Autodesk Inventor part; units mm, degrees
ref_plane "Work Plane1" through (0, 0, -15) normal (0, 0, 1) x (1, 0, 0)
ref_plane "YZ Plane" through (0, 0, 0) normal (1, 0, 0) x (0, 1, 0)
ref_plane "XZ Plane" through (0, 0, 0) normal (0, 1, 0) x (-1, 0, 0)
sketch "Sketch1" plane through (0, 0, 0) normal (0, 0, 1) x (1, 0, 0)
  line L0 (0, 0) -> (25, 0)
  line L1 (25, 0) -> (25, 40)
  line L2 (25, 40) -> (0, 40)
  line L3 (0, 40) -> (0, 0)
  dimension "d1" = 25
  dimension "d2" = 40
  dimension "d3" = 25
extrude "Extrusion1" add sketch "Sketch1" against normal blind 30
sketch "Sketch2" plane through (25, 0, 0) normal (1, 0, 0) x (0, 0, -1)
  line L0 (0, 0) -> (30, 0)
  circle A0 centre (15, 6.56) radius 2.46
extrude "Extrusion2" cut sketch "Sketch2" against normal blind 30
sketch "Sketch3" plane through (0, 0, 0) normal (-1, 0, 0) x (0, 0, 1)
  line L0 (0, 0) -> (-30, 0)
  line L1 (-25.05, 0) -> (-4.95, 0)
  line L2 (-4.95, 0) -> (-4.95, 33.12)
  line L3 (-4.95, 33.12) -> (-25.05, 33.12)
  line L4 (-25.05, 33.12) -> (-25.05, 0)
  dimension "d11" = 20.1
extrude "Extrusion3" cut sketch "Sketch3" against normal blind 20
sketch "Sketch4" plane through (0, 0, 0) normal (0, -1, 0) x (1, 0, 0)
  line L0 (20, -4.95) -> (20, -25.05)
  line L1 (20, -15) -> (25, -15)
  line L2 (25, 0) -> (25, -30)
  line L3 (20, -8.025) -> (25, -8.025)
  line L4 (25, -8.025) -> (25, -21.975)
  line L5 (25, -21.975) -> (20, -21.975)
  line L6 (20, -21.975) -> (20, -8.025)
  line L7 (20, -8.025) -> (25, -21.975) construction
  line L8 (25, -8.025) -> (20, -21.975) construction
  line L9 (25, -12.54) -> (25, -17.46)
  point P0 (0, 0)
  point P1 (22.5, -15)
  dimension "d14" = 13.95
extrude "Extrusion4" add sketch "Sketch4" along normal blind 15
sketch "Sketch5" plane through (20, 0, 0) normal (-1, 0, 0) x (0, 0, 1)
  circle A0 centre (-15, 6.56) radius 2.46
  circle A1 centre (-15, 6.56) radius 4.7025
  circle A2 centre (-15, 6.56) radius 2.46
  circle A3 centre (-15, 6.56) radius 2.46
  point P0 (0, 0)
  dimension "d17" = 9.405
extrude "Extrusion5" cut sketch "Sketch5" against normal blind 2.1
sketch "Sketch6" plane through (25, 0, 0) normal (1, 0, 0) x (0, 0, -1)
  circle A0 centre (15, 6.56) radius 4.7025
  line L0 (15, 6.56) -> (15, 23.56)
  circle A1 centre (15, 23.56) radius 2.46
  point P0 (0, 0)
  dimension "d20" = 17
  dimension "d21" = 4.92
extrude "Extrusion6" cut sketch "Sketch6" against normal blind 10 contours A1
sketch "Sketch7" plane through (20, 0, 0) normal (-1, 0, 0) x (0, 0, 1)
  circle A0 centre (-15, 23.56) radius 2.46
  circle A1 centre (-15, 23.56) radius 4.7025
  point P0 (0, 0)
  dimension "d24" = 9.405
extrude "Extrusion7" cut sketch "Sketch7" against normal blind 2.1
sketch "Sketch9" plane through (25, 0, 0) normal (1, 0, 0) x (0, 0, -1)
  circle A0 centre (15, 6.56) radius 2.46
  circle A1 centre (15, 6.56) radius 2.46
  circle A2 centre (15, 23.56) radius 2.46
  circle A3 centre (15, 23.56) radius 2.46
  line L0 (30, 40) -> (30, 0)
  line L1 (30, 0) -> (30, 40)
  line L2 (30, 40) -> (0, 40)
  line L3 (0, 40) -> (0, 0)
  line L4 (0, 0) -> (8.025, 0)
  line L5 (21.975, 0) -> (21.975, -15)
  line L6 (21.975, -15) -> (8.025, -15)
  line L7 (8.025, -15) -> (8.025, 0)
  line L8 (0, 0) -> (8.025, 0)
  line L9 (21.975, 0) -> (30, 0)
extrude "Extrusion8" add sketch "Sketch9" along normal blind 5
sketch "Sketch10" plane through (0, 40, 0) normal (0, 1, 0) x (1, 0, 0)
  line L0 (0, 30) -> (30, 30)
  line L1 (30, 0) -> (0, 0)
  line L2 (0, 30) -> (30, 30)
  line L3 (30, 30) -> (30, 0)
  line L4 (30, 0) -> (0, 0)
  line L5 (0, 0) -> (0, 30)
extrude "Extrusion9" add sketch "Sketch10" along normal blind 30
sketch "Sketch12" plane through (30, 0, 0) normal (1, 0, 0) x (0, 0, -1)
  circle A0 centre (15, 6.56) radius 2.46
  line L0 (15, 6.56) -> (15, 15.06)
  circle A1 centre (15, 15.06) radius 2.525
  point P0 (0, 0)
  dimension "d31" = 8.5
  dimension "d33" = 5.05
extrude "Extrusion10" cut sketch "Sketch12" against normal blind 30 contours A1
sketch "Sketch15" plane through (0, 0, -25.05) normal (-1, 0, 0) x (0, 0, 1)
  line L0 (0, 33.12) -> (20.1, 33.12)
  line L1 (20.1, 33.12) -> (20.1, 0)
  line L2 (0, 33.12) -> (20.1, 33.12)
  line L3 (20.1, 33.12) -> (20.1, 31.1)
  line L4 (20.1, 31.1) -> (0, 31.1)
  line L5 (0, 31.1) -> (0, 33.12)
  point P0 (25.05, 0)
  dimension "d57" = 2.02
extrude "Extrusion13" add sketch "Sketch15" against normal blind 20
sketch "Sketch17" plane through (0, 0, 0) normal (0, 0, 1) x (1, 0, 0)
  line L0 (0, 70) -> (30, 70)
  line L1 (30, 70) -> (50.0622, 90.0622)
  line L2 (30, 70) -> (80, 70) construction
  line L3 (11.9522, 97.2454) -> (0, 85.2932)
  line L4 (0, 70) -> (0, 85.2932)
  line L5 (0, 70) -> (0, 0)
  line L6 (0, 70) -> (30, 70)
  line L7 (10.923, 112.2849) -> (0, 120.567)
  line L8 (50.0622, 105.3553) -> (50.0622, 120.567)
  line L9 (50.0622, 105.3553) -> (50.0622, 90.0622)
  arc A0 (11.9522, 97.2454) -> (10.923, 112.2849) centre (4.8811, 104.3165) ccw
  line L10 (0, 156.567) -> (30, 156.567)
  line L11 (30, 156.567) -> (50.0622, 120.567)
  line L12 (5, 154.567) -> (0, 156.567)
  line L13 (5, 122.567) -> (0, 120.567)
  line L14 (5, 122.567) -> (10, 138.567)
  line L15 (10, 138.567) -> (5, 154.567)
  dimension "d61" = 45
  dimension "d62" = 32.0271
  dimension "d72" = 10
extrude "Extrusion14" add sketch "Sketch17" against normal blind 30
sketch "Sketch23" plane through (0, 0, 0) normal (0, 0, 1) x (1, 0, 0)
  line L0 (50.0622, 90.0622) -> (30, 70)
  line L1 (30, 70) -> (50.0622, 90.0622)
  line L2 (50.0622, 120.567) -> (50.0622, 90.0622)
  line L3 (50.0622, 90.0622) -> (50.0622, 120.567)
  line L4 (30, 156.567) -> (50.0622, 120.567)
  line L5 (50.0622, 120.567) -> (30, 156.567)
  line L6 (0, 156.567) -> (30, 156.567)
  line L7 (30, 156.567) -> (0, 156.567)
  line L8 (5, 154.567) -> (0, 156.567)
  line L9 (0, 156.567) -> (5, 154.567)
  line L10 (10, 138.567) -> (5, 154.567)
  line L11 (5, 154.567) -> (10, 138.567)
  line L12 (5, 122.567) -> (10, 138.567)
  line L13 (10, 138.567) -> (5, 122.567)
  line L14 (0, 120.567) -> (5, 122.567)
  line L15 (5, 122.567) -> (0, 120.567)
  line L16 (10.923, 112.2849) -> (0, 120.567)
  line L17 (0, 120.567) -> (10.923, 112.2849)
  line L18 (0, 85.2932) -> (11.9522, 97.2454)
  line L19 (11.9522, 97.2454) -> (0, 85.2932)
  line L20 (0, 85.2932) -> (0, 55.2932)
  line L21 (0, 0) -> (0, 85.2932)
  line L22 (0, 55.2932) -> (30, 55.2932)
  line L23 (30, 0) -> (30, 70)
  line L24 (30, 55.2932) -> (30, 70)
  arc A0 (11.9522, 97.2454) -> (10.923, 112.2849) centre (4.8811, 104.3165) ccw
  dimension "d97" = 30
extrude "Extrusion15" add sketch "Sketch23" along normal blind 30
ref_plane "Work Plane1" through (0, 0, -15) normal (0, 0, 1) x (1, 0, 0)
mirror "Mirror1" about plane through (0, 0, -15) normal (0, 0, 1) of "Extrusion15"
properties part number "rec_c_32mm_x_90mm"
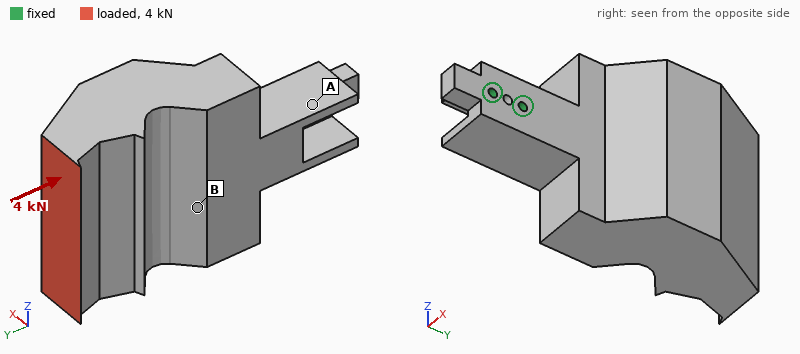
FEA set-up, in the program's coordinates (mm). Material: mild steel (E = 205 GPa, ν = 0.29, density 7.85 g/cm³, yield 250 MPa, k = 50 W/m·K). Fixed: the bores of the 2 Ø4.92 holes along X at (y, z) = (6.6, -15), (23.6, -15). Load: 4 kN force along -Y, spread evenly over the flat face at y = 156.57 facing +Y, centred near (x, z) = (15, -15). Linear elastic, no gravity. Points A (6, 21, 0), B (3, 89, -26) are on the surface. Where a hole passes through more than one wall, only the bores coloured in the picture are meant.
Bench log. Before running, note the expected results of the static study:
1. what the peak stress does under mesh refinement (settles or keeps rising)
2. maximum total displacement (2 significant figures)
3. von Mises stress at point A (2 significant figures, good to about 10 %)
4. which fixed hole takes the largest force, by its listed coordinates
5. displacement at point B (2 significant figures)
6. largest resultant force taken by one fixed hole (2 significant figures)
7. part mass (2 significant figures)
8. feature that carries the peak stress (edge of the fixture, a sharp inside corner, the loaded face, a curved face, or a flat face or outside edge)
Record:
keeps rising
46 µm
11 MPa
(23.6, -15)
21 µm
3.0 kN
2.9 kg
edge of the fixture
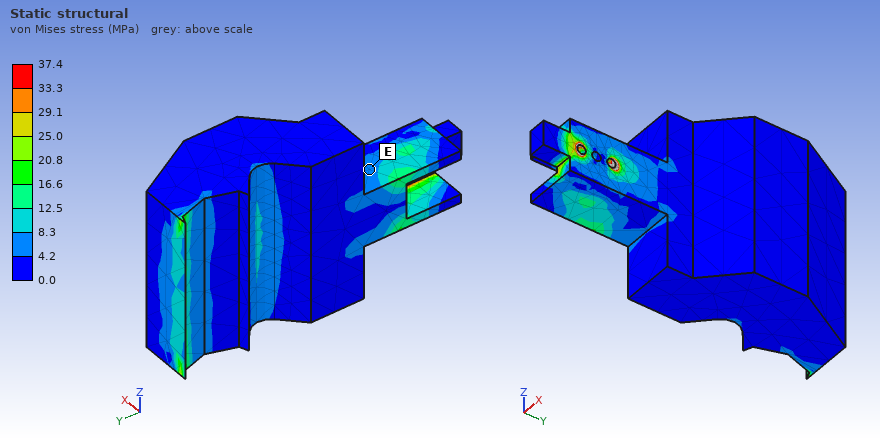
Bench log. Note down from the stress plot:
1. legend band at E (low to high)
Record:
4.2 to 8.3 MPa
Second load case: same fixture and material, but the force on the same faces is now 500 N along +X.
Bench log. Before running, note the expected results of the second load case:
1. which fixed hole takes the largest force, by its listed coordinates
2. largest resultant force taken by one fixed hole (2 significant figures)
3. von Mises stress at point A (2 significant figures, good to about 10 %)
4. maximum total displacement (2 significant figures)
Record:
(23.6, -15)
3.2 kN
18 MPa
85 µm
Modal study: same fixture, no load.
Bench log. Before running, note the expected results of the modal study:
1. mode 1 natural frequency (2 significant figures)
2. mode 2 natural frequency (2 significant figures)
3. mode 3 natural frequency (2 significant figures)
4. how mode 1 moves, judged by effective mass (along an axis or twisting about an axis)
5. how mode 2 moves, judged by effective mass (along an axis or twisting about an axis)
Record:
380 Hz
420 Hz
790 Hz
along X
along Z
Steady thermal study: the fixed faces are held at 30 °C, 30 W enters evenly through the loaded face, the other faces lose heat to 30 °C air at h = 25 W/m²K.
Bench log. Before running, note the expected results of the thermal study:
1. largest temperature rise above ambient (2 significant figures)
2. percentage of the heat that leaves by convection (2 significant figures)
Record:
37 K
63 %
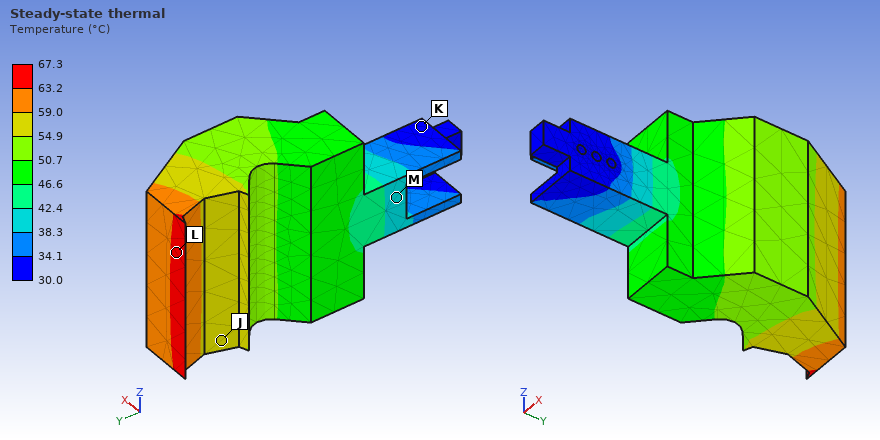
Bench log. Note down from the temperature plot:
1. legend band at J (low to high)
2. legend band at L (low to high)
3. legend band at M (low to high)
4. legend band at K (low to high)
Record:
54.9 to 59.0 °C
63.2 to 67.3 °C
38.3 to 42.4 °C
30.0 to 34.1 °C
